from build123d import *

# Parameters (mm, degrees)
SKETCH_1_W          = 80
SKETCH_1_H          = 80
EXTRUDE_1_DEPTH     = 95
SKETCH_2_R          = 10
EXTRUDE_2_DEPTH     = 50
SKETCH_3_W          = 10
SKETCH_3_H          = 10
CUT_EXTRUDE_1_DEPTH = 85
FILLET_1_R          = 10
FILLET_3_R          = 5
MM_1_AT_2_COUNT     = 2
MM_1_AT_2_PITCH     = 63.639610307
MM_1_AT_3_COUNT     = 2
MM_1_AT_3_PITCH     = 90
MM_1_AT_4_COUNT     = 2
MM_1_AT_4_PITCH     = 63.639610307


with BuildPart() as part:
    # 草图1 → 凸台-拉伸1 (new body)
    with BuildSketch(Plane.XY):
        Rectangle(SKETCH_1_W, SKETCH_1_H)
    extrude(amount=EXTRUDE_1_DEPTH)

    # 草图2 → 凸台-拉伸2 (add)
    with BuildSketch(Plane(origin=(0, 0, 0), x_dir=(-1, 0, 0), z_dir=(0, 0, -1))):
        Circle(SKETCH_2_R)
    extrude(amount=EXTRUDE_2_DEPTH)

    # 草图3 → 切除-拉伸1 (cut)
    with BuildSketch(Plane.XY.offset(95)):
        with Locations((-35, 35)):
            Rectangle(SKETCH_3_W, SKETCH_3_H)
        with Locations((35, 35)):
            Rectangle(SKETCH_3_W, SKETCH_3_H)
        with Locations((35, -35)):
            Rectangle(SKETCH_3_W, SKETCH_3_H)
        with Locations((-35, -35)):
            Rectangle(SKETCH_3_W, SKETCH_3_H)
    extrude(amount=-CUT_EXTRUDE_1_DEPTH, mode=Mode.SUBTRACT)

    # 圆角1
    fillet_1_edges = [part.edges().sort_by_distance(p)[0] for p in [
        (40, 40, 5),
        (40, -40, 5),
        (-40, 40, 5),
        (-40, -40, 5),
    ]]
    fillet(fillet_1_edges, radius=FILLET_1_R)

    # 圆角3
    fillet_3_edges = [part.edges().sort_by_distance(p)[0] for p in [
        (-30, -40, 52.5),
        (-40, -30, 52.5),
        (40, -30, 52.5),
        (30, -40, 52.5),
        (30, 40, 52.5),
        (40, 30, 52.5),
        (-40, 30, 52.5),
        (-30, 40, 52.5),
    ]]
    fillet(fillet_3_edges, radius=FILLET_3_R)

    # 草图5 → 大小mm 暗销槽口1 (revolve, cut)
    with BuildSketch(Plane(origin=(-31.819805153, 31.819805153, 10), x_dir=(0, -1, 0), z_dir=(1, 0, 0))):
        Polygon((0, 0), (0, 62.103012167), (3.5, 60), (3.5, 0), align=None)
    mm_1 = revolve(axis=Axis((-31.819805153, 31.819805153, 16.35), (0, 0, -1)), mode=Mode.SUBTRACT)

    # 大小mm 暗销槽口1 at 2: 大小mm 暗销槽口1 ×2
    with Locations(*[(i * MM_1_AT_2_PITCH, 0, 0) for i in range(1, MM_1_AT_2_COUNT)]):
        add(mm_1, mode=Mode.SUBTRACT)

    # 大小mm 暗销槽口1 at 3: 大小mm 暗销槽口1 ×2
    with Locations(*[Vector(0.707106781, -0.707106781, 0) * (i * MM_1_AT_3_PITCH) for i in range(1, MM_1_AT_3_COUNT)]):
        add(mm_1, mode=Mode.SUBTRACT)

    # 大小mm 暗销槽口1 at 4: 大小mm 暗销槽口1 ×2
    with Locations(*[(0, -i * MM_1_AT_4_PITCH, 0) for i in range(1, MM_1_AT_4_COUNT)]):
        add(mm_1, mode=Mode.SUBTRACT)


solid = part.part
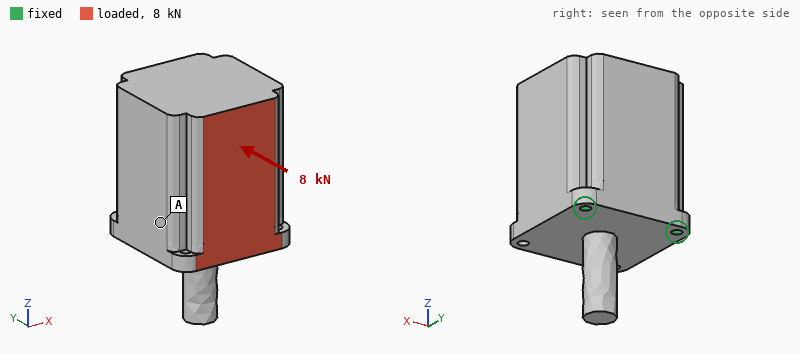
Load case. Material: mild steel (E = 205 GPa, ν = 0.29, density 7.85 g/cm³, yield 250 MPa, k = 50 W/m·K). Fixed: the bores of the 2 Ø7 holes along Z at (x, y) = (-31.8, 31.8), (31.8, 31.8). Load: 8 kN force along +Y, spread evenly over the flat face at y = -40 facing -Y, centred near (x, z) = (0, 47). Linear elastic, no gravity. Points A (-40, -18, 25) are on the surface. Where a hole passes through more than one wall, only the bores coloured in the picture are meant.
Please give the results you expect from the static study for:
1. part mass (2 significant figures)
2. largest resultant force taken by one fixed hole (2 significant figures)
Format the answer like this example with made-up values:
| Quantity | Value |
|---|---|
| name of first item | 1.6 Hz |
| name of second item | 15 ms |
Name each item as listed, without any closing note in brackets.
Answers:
| Quantity | Value |
|---|---|
| part mass | 4.6 kg |
| largest resultant force taken by one fixed hole | 4.1 kN |
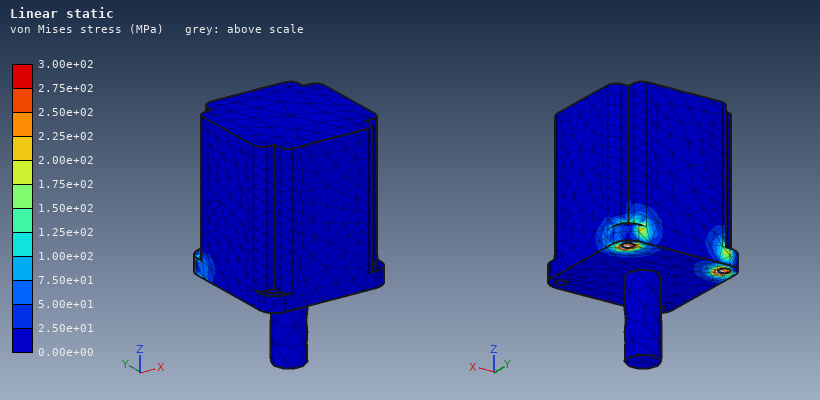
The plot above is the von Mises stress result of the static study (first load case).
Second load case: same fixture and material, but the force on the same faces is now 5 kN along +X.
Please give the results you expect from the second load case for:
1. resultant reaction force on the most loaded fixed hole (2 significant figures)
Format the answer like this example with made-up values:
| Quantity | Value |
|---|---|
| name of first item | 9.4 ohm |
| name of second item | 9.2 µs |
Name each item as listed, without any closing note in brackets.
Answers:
| Quantity | Value |
|---|---|
| resultant reaction force on the most loaded fixed hole | 6.9 kN |
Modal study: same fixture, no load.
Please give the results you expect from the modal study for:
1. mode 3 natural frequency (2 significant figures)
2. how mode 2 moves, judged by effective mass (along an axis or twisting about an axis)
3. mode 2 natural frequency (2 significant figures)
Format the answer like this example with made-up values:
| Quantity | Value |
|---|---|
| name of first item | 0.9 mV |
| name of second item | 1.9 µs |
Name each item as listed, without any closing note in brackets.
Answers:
| Quantity | Value |
|---|---|
| mode 3 natural frequency | 3800 Hz |
| how mode 2 moves, judged by effective mass | along X |
| mode 2 natural frequency | 2500 Hz |
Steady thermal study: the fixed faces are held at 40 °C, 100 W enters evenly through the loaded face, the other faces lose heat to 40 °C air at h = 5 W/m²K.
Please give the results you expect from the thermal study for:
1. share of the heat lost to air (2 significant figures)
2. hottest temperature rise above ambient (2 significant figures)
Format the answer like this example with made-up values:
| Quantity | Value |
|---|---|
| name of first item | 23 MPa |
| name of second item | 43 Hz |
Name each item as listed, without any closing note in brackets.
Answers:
| Quantity | Value |
|---|---|
| share of the heat lost to air | 8.3 % |
| hottest temperature rise above ambient | 59 K |
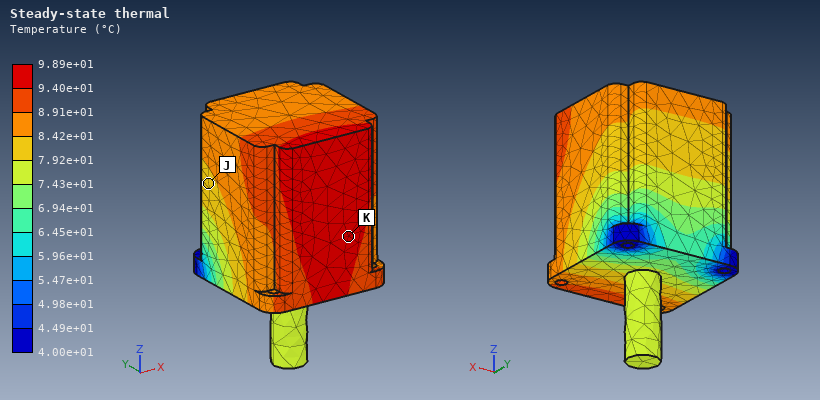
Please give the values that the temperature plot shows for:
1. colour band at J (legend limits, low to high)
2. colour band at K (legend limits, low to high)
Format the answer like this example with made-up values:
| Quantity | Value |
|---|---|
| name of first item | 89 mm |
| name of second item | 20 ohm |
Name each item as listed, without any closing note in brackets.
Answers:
| Quantity | Value |
|---|---|
| colour band at J | 7.92e+01 to 8.42e+01 °C |
| colour band at K | 9.40e+01 to 9.89e+01 °C |
